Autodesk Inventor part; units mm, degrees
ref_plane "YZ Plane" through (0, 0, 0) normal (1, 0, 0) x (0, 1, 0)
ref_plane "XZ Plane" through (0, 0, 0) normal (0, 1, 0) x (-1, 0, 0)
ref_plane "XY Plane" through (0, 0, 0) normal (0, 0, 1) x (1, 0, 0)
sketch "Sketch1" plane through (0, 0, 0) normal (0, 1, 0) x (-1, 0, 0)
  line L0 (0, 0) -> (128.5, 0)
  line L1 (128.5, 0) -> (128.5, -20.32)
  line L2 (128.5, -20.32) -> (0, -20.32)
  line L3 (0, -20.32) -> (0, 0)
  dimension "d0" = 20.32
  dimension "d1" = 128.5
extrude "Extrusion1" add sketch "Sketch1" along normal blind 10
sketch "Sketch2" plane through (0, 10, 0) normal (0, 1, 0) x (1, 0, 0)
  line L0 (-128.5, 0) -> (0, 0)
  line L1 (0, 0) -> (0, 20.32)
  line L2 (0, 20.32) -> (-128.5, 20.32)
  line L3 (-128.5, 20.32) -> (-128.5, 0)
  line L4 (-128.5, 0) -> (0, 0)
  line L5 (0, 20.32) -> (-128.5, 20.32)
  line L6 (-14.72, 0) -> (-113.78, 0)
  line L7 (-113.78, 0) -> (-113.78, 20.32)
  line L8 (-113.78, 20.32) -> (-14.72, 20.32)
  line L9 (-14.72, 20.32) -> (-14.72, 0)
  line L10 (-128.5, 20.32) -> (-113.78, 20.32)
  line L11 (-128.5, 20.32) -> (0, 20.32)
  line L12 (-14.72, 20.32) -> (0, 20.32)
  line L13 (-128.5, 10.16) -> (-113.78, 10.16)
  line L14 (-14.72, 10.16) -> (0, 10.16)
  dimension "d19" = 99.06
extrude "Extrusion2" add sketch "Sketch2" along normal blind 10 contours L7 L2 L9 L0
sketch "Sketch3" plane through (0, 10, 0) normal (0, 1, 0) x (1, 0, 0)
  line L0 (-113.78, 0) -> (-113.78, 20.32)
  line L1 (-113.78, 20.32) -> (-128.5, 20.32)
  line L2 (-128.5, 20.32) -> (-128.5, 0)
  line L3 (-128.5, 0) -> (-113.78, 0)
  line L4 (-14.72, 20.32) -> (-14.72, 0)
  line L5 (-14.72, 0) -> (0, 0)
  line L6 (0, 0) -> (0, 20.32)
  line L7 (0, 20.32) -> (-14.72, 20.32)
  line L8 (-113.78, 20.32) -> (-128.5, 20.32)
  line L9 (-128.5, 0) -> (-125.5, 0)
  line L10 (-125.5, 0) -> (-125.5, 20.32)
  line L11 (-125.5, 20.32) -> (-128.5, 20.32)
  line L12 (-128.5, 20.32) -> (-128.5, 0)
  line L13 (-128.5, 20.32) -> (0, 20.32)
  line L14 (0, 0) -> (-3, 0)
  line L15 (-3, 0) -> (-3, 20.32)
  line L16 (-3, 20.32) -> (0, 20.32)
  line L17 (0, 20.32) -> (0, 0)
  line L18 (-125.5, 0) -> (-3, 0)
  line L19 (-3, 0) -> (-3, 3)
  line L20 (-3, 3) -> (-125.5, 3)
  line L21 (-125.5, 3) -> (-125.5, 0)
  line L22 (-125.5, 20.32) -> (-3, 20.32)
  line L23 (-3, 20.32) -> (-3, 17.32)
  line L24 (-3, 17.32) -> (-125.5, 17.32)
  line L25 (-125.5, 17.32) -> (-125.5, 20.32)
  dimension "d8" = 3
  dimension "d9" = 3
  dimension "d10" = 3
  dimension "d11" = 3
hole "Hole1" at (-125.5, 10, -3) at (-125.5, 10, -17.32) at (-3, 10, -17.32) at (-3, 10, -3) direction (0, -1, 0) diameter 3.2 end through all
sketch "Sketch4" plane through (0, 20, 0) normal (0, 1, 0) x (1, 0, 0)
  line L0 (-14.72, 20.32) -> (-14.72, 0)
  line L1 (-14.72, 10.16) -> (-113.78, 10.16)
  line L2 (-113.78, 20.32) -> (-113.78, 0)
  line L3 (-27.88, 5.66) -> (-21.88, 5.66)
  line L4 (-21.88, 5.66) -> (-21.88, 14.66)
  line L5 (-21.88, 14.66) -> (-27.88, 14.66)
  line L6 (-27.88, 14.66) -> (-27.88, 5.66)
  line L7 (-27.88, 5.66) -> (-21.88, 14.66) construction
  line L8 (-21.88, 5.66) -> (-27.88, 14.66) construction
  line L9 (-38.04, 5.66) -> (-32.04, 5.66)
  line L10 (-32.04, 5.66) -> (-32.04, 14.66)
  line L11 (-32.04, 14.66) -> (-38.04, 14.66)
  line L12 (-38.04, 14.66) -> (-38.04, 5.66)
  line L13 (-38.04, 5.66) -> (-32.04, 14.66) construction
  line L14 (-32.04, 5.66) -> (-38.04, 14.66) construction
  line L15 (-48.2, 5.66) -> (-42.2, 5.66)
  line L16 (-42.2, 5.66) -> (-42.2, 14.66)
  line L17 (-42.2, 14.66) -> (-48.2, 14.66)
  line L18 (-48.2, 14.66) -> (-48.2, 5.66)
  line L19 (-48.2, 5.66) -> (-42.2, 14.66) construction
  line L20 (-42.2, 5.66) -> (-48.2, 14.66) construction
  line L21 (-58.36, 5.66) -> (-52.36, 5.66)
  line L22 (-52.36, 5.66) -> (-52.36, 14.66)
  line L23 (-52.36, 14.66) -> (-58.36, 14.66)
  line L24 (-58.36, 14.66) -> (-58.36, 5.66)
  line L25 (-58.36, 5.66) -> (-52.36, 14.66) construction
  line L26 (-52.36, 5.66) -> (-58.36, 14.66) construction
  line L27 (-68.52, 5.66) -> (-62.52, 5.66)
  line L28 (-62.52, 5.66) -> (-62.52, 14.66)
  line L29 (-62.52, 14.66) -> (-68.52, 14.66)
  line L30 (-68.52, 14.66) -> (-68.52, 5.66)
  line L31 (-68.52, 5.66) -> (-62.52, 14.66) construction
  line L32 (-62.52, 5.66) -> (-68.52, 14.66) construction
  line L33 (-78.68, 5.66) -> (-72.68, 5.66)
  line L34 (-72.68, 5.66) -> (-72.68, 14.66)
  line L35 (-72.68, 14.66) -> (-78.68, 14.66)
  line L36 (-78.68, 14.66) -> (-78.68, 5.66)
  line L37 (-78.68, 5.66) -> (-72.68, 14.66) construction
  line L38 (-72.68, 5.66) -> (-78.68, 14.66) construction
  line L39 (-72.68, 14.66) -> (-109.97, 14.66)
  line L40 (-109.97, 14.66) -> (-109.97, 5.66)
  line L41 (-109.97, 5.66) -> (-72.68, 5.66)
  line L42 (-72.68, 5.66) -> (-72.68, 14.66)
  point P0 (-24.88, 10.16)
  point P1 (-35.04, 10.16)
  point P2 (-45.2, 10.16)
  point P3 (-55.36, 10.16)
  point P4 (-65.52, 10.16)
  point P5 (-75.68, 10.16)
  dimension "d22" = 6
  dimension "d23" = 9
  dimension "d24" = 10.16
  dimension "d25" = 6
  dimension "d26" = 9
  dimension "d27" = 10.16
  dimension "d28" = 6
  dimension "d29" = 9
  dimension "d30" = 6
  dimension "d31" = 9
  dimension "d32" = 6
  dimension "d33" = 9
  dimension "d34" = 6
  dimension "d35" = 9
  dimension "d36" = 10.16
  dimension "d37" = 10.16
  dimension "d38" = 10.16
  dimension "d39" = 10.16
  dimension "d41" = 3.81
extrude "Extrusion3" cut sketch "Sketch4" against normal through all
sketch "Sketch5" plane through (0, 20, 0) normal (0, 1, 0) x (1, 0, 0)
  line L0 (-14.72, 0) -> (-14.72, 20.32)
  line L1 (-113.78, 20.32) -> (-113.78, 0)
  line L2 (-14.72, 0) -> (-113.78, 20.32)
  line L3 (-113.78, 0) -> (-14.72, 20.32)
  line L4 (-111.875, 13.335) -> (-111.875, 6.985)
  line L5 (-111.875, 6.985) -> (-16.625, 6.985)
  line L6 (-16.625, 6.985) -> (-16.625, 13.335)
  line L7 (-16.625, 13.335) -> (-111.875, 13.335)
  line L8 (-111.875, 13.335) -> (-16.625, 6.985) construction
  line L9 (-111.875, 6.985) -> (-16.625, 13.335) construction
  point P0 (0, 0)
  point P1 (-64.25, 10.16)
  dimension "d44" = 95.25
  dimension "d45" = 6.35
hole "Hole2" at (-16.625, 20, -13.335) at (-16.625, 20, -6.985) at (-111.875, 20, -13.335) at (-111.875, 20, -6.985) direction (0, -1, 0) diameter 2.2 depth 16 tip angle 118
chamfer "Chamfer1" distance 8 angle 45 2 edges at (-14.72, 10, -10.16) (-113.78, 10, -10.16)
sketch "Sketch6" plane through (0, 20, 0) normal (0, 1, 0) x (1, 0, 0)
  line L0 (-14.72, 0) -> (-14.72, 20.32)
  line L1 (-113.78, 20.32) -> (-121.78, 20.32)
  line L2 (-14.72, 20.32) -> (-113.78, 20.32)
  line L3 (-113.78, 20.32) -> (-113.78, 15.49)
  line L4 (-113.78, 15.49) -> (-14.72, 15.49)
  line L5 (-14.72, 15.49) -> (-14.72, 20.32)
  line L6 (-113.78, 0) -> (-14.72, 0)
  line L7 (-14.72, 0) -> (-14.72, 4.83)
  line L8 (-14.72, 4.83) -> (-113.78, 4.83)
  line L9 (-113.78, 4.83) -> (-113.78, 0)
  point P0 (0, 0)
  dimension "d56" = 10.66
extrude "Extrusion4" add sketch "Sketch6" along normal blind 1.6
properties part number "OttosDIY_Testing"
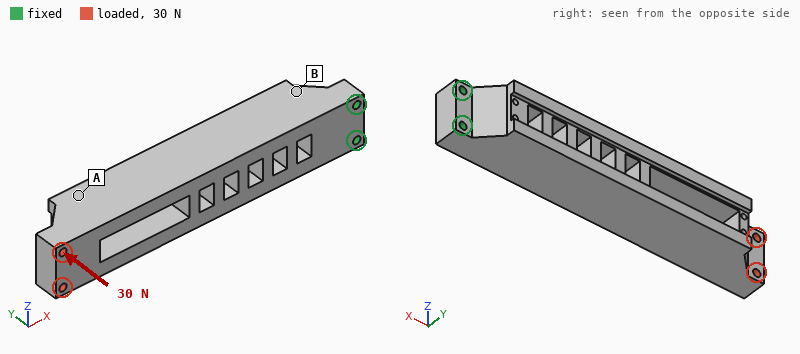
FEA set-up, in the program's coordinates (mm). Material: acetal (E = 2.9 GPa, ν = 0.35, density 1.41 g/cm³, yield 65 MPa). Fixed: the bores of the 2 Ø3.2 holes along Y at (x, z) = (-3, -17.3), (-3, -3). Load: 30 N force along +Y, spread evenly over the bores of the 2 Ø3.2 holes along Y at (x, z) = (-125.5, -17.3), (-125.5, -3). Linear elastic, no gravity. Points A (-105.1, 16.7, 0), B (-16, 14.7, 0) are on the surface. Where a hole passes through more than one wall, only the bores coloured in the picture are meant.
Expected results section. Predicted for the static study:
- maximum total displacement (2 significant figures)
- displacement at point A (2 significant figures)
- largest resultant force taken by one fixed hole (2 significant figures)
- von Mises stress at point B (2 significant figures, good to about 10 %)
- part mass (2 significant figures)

1.4 mm
1.1 mm
17 N
2.8 MPa
51 g
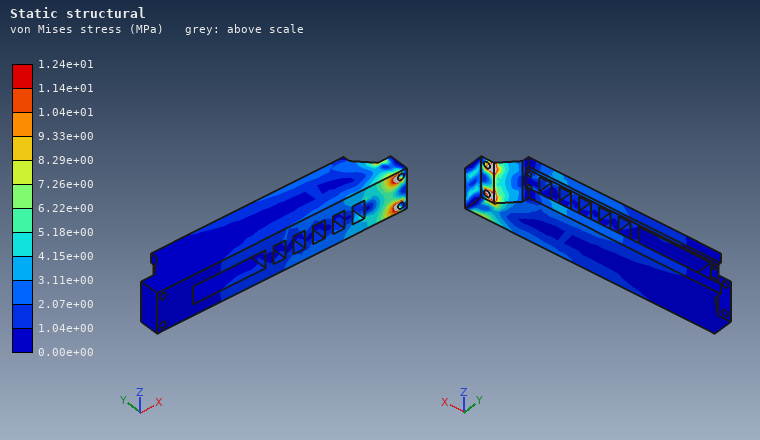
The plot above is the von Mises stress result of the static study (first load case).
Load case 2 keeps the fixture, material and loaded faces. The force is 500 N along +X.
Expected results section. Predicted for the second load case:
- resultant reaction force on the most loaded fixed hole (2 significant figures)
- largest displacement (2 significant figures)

250 N
0.73 mm
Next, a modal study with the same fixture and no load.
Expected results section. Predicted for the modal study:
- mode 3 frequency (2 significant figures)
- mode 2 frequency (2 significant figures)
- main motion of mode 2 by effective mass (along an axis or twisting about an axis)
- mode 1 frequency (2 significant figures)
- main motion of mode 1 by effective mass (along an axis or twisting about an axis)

1100 Hz
290 Hz
along Z
200 Hz
along Y
